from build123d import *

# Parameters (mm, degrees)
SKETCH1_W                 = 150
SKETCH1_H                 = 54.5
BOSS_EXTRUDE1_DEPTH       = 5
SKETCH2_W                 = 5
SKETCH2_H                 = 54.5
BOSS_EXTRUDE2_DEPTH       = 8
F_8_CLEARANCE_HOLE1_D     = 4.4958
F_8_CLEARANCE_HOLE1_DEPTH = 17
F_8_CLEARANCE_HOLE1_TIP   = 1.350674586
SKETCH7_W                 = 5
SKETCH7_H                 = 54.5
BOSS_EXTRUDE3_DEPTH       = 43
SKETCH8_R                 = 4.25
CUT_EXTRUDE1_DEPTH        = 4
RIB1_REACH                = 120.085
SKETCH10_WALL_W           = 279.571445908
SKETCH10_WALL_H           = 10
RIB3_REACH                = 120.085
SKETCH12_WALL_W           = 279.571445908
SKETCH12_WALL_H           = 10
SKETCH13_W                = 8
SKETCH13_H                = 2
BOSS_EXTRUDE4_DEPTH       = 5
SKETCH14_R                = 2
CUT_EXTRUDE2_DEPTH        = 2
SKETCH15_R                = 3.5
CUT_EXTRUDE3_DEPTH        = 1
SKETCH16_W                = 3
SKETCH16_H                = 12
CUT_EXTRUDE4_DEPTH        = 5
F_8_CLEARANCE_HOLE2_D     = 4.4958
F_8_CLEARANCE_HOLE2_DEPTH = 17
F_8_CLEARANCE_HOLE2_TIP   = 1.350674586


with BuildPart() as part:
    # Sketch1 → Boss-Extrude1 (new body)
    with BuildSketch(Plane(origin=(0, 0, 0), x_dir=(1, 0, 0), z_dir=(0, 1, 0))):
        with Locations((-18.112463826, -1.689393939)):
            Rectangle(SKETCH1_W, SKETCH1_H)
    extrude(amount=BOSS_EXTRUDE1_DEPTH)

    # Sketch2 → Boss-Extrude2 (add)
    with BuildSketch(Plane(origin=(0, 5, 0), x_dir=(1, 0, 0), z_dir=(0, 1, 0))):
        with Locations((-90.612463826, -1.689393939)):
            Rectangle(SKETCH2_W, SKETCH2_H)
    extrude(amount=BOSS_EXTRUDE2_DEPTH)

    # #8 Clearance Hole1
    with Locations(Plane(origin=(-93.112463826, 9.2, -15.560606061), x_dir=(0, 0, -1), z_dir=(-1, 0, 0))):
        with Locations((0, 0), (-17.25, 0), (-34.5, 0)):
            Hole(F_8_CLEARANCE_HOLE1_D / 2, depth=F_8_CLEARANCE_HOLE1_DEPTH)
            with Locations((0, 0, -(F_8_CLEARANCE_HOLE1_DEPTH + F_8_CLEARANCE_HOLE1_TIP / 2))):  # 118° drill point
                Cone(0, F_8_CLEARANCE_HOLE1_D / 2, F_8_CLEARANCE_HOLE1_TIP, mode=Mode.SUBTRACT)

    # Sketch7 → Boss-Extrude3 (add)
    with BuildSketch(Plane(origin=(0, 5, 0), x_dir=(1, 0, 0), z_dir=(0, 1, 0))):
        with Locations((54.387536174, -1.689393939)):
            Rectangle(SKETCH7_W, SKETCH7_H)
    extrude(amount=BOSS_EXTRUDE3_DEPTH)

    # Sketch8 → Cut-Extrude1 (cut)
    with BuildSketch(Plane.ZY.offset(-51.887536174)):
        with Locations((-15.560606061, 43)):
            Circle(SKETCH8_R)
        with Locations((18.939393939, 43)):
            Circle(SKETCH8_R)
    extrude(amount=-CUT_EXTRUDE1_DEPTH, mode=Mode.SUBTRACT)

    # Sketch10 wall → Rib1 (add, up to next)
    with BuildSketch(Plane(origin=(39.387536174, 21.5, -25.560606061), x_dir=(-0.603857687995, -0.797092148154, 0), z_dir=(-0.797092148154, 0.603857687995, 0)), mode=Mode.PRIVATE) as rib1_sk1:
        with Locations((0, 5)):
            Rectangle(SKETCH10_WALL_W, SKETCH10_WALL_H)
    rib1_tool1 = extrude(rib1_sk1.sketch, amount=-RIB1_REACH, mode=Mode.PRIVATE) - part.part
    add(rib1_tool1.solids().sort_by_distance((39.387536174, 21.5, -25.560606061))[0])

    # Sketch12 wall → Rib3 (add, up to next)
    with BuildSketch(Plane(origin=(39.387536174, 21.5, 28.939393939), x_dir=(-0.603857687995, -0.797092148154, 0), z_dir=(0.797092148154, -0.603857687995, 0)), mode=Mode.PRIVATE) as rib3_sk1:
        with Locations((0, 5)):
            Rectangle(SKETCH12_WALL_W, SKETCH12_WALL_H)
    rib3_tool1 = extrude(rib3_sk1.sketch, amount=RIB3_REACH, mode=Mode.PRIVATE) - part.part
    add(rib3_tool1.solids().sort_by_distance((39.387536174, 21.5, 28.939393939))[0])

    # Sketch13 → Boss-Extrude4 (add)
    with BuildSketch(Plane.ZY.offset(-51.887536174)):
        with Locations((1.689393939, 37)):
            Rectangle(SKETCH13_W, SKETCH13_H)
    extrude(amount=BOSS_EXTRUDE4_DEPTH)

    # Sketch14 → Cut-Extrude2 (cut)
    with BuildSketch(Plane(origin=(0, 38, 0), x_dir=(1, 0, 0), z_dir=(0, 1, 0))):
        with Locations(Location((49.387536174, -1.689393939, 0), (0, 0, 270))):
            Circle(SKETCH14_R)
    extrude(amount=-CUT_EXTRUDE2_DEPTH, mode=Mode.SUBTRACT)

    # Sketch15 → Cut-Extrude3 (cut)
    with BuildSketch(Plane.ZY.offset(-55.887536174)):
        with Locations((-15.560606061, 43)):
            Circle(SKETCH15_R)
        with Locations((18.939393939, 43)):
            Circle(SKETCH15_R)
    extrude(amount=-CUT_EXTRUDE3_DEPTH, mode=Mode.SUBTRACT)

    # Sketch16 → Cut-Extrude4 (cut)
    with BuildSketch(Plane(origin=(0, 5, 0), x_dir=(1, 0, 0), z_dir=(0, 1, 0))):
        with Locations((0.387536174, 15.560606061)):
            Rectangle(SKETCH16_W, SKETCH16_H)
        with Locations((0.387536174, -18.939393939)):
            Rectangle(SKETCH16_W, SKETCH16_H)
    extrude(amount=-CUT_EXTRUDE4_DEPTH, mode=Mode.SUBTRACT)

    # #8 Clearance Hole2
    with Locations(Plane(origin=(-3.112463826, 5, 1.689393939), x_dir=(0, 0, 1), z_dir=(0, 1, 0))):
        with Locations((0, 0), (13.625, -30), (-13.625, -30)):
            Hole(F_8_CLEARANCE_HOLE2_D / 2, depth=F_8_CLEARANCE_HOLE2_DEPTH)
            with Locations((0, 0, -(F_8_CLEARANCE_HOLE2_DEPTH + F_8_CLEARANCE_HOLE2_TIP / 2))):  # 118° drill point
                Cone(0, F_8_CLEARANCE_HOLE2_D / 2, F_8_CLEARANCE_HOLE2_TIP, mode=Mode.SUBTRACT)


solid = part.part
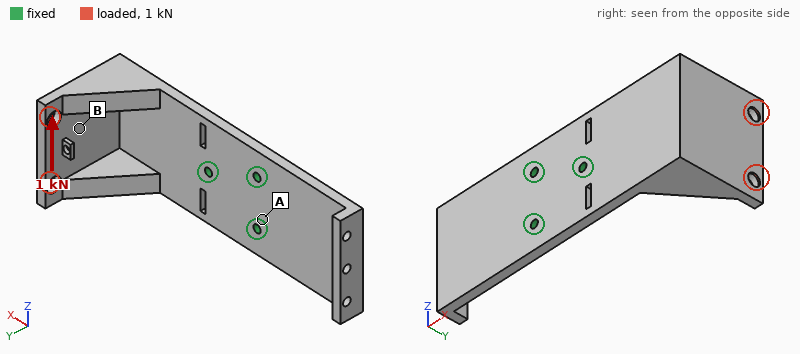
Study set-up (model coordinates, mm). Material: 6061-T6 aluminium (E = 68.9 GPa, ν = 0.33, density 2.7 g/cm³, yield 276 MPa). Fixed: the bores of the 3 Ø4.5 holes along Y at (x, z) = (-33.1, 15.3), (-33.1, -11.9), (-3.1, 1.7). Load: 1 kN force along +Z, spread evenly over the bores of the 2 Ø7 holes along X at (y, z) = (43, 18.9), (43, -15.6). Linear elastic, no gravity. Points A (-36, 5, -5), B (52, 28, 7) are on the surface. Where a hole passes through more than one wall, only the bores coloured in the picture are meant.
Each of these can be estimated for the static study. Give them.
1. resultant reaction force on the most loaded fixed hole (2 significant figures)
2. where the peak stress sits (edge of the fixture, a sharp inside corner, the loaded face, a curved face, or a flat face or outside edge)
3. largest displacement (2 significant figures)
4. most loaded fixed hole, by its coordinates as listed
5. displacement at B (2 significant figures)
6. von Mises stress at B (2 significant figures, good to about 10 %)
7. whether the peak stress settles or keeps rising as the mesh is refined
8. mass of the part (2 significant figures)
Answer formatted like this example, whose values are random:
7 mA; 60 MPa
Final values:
1.9 kN; edge of the fixture; 1.4 mm; (-3.1, 1.7); 0.71 mm; 38 MPa; keeps rising; 170 g
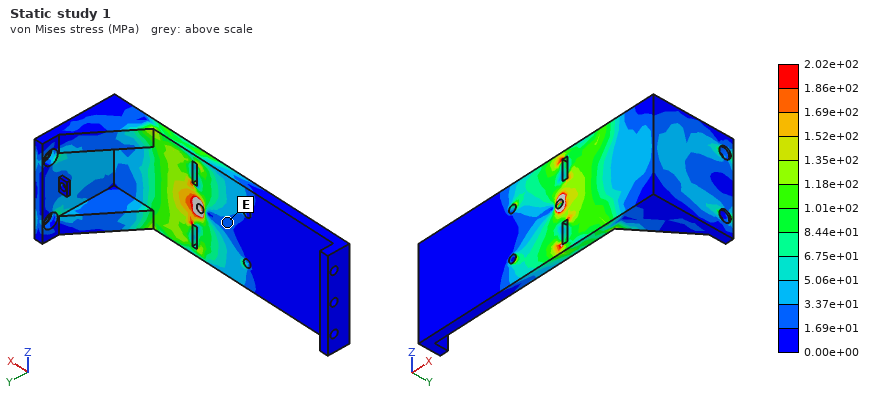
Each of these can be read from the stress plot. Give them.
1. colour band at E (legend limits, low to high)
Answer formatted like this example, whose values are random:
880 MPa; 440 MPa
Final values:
1.69e+01 to 3.37e+01 MPa
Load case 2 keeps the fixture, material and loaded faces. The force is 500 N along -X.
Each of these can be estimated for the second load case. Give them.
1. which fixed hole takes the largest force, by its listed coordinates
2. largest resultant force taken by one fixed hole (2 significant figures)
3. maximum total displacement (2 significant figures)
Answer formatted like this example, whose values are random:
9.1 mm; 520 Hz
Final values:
(-3.1, 1.7); 480 N; 1.4 mm
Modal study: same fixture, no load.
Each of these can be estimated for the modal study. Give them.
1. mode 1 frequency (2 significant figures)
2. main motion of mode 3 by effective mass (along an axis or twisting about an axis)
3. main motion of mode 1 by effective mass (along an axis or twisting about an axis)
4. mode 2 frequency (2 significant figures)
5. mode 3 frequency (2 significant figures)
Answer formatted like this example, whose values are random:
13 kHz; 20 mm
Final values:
430 Hz; along Y; along Y; 880 Hz; 950 Hz
